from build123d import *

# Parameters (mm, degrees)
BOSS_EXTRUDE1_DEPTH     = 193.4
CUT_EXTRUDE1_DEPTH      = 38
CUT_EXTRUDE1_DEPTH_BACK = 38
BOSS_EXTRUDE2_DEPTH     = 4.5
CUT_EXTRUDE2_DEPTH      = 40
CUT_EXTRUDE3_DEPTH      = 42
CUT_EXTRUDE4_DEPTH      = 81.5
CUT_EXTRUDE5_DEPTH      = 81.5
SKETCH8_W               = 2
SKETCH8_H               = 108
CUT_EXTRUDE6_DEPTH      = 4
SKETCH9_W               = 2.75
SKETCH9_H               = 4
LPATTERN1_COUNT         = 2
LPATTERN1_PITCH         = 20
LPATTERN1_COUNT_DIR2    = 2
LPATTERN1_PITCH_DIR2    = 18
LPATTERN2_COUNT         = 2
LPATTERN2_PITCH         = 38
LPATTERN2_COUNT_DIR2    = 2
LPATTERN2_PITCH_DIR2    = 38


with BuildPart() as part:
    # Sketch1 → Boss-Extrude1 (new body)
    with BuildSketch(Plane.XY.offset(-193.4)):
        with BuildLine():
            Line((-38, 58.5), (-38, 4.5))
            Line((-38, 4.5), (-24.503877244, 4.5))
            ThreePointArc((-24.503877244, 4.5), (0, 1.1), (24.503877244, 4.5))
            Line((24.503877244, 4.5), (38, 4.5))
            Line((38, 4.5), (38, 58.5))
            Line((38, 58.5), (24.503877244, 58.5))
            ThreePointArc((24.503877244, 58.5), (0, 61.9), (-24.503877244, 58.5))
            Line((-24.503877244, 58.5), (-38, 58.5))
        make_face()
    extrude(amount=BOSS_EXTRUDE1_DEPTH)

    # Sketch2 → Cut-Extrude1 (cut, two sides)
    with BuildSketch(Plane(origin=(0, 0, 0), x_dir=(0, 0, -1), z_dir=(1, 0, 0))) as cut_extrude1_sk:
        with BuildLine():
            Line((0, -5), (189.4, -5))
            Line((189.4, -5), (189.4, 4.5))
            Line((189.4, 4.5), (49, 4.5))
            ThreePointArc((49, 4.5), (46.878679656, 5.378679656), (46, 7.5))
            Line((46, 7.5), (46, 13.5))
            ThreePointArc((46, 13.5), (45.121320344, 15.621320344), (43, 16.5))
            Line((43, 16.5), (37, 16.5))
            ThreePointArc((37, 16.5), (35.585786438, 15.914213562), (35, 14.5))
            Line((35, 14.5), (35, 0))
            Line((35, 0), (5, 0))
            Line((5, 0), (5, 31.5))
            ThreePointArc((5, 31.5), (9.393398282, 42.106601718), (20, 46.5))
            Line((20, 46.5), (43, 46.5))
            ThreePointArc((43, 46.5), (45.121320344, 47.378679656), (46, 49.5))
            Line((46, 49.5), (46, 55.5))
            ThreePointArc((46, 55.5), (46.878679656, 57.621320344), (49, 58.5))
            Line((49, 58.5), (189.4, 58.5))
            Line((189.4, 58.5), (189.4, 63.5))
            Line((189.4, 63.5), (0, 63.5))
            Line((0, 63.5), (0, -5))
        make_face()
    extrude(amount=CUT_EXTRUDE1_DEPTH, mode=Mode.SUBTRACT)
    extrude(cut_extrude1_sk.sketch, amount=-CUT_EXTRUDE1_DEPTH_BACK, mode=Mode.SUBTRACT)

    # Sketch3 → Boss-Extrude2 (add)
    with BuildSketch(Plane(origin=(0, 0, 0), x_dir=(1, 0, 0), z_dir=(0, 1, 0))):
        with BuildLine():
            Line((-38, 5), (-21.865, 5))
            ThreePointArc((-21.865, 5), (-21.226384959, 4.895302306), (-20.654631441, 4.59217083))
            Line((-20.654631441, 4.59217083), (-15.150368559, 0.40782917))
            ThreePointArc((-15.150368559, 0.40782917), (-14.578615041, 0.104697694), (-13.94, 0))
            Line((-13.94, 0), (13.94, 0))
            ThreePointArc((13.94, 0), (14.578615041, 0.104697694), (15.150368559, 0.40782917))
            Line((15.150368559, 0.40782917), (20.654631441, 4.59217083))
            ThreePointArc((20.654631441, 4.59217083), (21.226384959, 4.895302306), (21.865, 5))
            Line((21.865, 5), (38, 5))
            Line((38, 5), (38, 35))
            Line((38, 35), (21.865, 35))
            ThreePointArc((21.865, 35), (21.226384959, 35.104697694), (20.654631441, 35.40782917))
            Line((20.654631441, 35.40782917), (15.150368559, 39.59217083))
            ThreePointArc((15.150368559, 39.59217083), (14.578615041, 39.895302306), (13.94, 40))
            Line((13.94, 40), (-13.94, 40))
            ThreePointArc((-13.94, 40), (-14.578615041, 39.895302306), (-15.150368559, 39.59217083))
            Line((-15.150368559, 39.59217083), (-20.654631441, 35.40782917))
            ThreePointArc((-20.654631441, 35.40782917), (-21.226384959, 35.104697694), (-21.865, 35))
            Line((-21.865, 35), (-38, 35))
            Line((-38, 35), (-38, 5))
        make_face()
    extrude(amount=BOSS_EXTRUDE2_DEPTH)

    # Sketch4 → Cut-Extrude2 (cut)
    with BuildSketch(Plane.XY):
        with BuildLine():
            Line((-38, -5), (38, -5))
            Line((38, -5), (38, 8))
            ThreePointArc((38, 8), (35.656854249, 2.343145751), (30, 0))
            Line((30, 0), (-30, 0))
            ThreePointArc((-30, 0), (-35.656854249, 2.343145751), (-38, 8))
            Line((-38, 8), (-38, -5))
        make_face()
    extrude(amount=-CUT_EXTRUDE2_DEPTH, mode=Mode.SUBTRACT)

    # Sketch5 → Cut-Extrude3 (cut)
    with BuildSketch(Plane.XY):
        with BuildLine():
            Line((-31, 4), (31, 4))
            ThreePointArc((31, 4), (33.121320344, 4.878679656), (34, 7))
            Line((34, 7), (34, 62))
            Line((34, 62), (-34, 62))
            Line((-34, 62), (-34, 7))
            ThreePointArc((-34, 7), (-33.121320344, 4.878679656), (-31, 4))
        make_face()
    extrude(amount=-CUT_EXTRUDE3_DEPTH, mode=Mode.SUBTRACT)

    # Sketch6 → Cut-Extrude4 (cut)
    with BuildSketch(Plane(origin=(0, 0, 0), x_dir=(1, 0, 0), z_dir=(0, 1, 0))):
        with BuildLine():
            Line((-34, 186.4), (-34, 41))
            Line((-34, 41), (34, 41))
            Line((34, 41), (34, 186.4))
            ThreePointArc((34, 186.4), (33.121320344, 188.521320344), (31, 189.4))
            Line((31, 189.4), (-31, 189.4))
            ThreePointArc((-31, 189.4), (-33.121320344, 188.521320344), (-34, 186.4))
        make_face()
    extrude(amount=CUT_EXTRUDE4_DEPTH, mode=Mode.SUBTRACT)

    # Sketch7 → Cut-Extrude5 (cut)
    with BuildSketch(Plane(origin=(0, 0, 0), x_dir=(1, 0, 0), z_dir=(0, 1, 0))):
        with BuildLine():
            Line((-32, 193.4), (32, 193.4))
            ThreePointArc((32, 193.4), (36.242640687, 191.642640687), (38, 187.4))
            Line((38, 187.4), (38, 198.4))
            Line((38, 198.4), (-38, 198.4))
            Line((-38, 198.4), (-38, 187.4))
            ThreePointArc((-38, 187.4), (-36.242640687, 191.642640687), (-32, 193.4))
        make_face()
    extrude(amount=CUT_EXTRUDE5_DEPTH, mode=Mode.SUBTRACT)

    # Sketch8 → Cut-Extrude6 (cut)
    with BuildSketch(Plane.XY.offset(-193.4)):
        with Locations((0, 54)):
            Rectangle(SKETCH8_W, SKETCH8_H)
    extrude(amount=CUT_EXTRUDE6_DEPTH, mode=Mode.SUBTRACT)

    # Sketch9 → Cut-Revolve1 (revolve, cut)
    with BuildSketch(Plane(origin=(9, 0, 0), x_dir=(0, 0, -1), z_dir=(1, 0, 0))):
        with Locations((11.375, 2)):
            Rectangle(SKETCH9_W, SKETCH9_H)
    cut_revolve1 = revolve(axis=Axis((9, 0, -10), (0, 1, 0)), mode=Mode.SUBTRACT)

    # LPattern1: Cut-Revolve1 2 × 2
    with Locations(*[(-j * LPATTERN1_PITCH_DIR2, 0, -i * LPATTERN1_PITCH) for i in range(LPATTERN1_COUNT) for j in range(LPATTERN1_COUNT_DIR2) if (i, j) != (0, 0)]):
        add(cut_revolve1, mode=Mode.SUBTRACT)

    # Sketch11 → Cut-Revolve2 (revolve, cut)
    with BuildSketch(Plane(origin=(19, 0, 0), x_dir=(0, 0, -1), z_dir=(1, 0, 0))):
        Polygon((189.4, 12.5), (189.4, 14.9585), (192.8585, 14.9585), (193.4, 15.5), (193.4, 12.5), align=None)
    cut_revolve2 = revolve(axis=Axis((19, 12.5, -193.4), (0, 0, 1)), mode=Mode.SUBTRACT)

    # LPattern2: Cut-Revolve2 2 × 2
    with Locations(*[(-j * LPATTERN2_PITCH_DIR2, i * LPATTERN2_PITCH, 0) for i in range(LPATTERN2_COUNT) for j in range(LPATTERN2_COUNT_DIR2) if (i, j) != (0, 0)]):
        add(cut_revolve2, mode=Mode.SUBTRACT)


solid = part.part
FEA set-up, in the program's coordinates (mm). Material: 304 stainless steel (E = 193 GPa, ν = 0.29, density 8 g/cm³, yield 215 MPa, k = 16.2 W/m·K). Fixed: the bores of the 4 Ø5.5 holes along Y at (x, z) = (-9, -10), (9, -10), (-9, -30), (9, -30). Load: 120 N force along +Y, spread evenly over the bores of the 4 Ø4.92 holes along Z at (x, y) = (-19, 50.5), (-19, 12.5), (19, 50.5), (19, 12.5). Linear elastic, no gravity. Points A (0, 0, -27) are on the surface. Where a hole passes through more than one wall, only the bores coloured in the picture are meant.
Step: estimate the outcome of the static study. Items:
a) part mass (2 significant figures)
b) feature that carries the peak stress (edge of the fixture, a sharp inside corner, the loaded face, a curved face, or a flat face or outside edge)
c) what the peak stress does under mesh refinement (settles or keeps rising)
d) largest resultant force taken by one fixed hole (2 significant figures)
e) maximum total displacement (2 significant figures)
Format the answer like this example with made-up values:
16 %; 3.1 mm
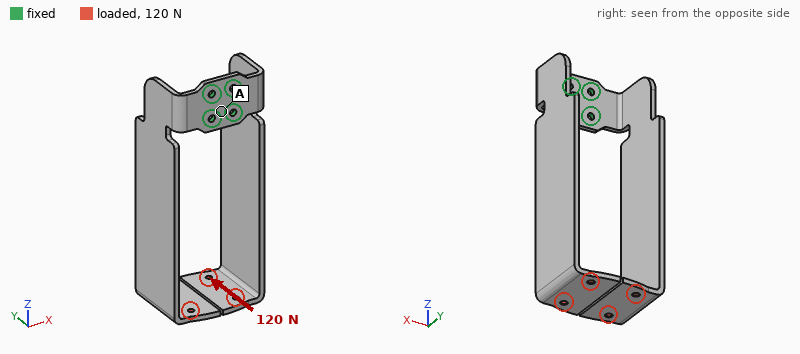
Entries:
800 g; edge of the fixture; keeps rising; 460 N; 0.79 mm
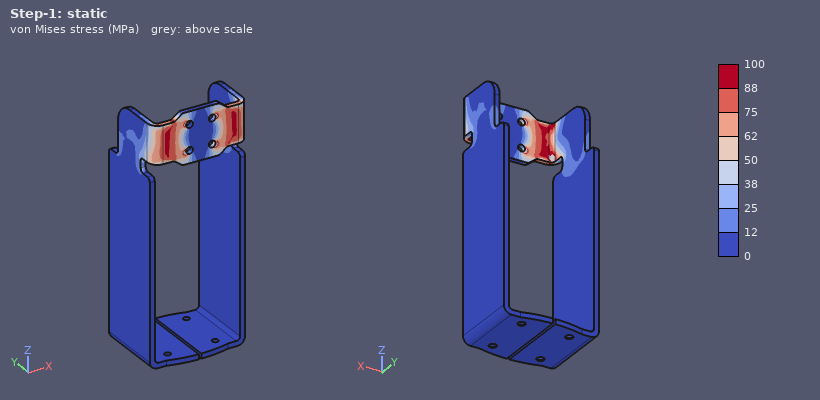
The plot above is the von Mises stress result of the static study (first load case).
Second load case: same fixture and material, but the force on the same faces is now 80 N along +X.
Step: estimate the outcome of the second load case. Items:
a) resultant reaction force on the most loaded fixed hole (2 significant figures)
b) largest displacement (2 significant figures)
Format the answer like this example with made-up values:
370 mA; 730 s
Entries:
310 N; 2.1 mm
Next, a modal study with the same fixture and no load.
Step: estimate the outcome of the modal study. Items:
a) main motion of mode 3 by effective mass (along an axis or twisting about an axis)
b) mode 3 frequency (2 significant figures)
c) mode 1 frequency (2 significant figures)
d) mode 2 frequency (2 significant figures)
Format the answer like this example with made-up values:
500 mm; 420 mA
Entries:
along Y; 120 Hz; 60 Hz; 60 Hz
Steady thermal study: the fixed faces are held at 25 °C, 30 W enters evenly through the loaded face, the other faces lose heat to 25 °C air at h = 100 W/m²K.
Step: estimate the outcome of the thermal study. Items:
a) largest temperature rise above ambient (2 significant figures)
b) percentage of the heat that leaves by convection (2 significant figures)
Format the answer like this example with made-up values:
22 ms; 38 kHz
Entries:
57 K; 100 %
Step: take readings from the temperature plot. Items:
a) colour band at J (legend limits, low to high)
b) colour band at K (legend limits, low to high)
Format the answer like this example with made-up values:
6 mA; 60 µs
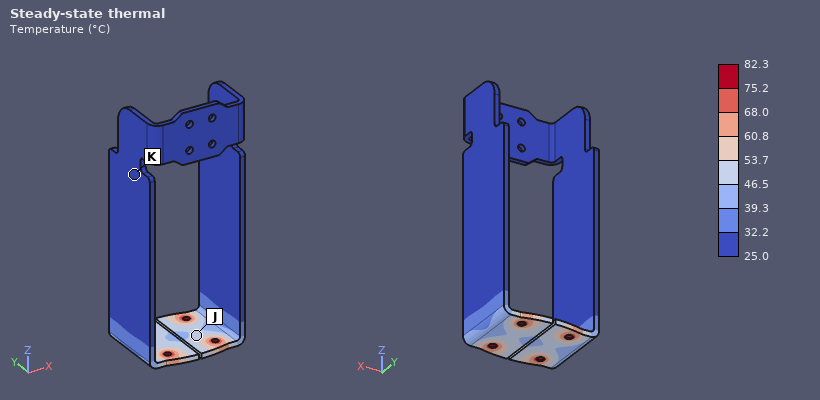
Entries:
46.5 to 53.7 °C; 25.0 to 32.2 °C
